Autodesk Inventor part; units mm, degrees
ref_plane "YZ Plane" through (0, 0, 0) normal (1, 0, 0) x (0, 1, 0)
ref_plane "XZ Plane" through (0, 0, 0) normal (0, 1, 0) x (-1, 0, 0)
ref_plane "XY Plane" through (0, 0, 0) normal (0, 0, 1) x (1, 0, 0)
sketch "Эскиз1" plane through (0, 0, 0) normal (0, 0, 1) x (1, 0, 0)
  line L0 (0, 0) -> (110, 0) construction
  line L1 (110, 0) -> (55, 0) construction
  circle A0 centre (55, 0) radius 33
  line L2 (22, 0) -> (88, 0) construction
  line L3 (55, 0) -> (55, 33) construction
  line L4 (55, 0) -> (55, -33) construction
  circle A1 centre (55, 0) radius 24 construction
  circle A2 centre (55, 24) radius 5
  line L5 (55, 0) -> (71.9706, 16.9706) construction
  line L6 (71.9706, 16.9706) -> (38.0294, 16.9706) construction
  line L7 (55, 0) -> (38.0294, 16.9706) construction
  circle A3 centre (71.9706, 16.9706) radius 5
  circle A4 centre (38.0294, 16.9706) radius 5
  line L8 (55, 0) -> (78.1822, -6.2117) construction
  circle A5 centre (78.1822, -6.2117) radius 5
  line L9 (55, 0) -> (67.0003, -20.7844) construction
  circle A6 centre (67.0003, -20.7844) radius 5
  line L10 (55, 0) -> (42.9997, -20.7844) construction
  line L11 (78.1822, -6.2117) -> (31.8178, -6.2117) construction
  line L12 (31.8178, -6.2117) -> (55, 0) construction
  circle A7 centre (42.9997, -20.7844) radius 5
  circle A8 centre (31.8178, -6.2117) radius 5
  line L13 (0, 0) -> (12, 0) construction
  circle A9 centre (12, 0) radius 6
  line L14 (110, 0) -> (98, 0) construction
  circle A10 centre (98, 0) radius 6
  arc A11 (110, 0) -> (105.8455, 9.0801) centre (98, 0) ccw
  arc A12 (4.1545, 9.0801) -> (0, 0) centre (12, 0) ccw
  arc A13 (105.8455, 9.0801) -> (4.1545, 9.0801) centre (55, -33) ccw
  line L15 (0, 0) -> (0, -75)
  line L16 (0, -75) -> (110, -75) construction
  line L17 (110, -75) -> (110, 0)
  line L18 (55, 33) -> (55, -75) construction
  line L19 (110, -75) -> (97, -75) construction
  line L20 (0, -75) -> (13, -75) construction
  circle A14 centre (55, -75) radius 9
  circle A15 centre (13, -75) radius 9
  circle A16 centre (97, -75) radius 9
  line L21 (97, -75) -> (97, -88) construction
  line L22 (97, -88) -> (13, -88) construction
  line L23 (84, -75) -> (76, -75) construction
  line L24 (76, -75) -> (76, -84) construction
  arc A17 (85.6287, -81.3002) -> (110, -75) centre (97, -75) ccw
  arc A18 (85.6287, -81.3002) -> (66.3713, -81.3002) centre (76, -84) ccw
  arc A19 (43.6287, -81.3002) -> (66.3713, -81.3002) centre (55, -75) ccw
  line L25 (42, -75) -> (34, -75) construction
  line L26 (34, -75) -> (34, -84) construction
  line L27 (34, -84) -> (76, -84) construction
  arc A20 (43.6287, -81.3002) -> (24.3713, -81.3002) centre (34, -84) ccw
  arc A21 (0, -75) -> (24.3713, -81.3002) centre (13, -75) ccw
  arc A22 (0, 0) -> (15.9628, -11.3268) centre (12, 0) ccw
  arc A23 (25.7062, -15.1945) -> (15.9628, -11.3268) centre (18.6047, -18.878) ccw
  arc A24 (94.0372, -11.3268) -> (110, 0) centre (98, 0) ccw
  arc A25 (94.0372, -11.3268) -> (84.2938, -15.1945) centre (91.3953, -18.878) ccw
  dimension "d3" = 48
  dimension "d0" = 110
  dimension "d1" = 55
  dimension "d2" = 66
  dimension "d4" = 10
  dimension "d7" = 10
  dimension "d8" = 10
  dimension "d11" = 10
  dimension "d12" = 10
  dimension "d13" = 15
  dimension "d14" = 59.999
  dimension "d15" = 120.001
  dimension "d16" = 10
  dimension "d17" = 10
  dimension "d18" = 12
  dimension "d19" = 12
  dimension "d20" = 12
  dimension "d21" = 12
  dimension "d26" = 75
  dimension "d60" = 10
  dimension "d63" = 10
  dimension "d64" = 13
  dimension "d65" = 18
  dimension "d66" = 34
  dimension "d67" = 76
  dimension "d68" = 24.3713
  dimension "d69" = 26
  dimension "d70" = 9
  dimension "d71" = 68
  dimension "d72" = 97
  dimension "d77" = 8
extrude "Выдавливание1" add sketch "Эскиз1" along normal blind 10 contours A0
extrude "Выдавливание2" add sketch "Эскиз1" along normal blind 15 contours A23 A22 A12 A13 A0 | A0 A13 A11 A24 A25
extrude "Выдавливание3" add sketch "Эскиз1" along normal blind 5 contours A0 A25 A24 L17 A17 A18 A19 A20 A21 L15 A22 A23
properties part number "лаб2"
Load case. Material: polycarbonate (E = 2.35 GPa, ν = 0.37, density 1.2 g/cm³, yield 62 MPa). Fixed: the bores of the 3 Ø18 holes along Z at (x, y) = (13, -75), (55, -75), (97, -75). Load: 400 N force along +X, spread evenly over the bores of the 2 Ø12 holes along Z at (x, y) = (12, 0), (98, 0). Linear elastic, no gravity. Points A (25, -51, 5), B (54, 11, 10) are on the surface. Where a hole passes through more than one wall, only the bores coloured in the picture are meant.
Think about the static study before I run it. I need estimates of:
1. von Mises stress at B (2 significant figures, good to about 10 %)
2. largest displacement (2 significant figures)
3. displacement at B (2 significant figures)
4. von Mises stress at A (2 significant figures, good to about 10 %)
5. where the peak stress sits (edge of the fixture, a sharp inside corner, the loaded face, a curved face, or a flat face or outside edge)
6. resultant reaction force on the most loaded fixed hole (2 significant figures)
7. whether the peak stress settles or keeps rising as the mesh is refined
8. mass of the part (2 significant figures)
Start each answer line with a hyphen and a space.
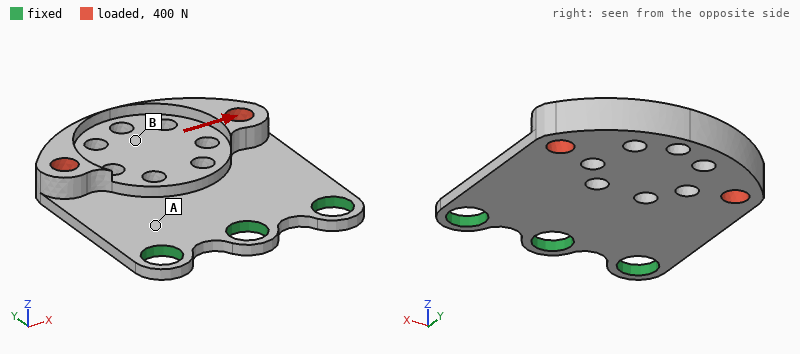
- 0.57 MPa
- 0.47 mm
- 0.15 mm
- 2.7 MPa
- edge of the fixture
- 340 N
- keeps rising
- 93 g
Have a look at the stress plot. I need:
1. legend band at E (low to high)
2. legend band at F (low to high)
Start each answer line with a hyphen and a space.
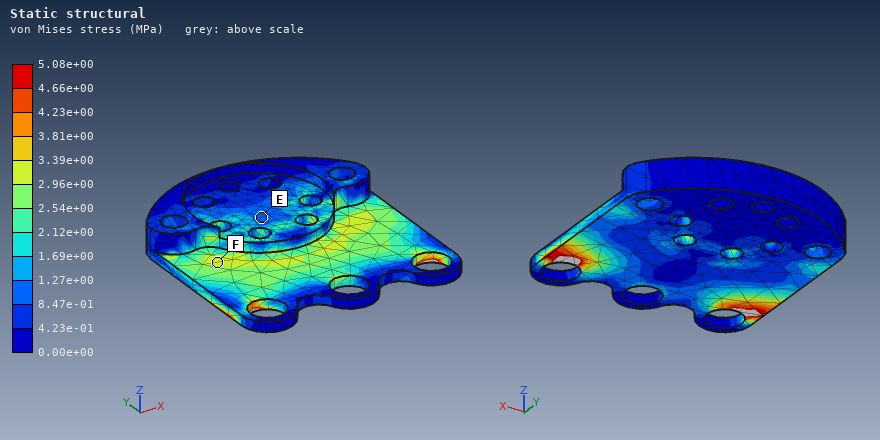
- 8.47e-01 to 1.27e+00 MPa
- 2.96e+00 to 3.39e+00 MPa
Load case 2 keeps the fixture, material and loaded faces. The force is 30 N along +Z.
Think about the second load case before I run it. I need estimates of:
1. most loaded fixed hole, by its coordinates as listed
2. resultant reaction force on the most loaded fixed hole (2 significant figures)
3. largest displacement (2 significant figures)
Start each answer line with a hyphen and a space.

- (55, -75)
- 13 N
- 1.7 mm
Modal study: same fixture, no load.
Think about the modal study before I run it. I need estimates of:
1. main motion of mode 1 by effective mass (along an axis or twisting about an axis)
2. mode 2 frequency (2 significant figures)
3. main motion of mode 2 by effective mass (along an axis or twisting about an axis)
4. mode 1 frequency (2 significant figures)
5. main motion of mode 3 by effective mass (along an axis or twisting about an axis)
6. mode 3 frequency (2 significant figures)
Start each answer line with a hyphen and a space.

- along Z
- 320 Hz
- twisting about Y
- 100 Hz
- along Z
- 820 Hz
